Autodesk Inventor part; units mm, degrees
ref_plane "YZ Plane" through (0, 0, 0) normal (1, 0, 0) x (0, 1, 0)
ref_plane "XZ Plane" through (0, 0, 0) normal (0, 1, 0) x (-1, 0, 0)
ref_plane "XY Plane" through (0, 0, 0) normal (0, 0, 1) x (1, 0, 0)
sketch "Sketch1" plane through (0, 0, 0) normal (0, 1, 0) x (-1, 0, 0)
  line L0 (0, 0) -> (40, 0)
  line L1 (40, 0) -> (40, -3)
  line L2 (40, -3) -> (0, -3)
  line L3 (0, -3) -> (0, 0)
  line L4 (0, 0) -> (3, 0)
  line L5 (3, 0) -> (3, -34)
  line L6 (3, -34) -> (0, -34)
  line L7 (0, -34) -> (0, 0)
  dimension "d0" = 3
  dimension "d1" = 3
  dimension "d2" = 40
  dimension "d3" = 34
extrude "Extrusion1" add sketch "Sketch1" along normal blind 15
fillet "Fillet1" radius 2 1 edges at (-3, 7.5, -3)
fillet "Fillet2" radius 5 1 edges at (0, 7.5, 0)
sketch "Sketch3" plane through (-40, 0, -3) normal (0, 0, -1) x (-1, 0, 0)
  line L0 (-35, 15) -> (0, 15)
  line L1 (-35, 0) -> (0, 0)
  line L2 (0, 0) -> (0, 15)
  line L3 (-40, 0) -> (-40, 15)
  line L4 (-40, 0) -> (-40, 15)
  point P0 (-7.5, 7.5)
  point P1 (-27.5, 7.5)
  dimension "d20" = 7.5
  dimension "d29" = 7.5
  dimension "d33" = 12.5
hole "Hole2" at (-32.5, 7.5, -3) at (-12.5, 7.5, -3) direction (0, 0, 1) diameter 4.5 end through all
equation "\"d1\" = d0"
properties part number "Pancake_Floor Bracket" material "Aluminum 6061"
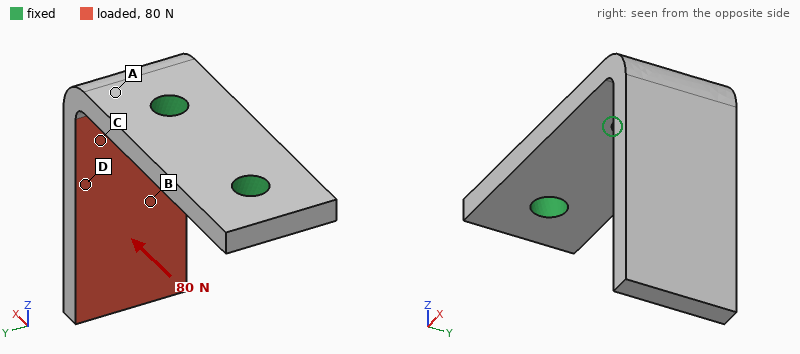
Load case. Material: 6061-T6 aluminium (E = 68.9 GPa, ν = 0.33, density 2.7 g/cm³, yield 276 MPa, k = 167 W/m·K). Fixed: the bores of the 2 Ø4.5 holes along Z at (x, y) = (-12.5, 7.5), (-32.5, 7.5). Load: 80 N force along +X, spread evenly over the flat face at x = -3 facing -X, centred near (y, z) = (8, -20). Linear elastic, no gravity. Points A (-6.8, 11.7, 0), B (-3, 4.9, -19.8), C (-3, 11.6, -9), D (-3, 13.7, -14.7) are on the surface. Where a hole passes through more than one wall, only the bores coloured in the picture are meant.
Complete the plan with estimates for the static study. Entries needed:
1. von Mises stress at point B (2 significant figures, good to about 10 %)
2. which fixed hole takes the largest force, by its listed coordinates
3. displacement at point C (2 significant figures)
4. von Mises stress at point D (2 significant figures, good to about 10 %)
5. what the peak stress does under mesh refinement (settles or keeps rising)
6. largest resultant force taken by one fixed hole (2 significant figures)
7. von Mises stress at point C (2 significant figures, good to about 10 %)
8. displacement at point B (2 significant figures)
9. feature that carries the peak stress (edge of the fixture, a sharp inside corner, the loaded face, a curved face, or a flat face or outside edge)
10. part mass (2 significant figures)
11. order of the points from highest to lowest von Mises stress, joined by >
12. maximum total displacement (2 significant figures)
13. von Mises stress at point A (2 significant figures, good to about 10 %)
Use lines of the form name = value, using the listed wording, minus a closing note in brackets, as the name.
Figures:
von Mises stress at point B = 13 MPa
which fixed hole takes the largest force, by its listed coordinates = (-12.5, 7.5)
displacement at point C = 0.055 mm
von Mises stress at point D = 23 MPa
what the peak stress does under mesh refinement = keeps rising
largest resultant force taken by one fixed hole = 75 N
von Mises stress at point C = 37 MPa
displacement at point B = 0.16 mm
feature that carries the peak stress = edge of the fixture
part mass = 8.2 g
order of the points from highest to lowest von Mises stress, joined by > = A > C > D > B
maximum total displacement = 0.33 mm
von Mises stress at point A = 56 MPa
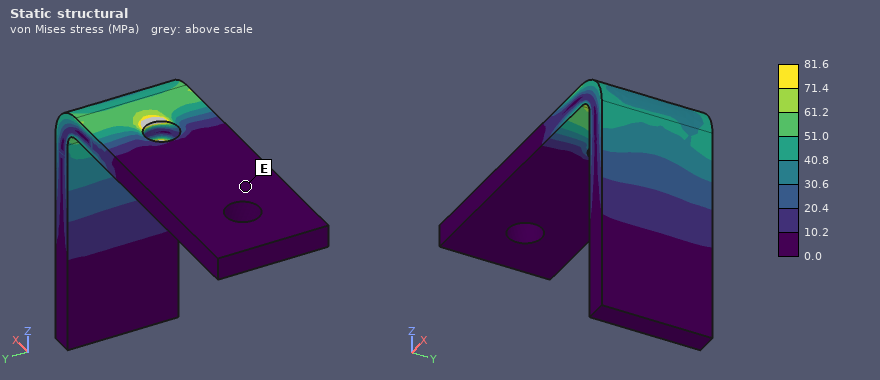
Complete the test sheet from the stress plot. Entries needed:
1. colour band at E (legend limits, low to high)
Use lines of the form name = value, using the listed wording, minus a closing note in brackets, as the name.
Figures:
colour band at E = 0.0 to 10.2 MPa
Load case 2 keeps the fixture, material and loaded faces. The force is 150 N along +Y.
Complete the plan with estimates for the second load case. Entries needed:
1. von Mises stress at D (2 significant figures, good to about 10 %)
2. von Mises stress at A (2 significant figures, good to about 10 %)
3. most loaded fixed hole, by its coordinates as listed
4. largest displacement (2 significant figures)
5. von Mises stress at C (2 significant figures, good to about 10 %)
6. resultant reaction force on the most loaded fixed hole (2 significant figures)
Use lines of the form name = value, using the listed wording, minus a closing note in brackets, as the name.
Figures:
von Mises stress at D = 14 MPa
von Mises stress at A = 66 MPa
most loaded fixed hole, by its coordinates as listed = (-12.5, 7.5)
largest displacement = 0.23 mm
von Mises stress at C = 29 MPa
resultant reaction force on the most loaded fixed hole = 180 N
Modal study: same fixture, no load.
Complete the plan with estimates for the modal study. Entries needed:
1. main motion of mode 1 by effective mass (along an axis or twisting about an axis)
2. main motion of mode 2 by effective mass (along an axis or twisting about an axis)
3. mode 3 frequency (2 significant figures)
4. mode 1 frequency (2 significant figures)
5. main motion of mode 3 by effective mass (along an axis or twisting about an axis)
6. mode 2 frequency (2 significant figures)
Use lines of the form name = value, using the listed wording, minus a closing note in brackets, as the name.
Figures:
main motion of mode 1 by effective mass = along X
main motion of mode 2 by effective mass = along Y
mode 3 frequency = 7800 Hz
mode 1 frequency = 1600 Hz
main motion of mode 3 by effective mass = along Z
mode 2 frequency = 2600 Hz
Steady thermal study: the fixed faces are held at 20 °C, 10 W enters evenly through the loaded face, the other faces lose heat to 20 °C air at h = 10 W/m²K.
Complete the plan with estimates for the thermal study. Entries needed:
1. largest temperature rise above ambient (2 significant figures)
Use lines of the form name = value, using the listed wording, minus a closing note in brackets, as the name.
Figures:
largest temperature rise above ambient = 35 K
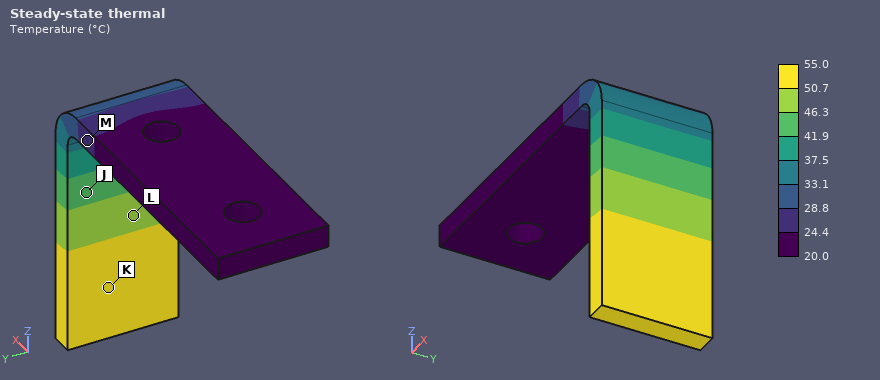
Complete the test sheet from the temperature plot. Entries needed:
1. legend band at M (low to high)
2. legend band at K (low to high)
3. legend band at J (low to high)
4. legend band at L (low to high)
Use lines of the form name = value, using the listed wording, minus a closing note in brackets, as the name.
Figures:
legend band at M = 24.4 to 28.8 °C
legend band at K = 50.7 to 55.0 °C
legend band at J = 41.9 to 46.3 °C
legend band at L = 46.3 to 50.7 °C
